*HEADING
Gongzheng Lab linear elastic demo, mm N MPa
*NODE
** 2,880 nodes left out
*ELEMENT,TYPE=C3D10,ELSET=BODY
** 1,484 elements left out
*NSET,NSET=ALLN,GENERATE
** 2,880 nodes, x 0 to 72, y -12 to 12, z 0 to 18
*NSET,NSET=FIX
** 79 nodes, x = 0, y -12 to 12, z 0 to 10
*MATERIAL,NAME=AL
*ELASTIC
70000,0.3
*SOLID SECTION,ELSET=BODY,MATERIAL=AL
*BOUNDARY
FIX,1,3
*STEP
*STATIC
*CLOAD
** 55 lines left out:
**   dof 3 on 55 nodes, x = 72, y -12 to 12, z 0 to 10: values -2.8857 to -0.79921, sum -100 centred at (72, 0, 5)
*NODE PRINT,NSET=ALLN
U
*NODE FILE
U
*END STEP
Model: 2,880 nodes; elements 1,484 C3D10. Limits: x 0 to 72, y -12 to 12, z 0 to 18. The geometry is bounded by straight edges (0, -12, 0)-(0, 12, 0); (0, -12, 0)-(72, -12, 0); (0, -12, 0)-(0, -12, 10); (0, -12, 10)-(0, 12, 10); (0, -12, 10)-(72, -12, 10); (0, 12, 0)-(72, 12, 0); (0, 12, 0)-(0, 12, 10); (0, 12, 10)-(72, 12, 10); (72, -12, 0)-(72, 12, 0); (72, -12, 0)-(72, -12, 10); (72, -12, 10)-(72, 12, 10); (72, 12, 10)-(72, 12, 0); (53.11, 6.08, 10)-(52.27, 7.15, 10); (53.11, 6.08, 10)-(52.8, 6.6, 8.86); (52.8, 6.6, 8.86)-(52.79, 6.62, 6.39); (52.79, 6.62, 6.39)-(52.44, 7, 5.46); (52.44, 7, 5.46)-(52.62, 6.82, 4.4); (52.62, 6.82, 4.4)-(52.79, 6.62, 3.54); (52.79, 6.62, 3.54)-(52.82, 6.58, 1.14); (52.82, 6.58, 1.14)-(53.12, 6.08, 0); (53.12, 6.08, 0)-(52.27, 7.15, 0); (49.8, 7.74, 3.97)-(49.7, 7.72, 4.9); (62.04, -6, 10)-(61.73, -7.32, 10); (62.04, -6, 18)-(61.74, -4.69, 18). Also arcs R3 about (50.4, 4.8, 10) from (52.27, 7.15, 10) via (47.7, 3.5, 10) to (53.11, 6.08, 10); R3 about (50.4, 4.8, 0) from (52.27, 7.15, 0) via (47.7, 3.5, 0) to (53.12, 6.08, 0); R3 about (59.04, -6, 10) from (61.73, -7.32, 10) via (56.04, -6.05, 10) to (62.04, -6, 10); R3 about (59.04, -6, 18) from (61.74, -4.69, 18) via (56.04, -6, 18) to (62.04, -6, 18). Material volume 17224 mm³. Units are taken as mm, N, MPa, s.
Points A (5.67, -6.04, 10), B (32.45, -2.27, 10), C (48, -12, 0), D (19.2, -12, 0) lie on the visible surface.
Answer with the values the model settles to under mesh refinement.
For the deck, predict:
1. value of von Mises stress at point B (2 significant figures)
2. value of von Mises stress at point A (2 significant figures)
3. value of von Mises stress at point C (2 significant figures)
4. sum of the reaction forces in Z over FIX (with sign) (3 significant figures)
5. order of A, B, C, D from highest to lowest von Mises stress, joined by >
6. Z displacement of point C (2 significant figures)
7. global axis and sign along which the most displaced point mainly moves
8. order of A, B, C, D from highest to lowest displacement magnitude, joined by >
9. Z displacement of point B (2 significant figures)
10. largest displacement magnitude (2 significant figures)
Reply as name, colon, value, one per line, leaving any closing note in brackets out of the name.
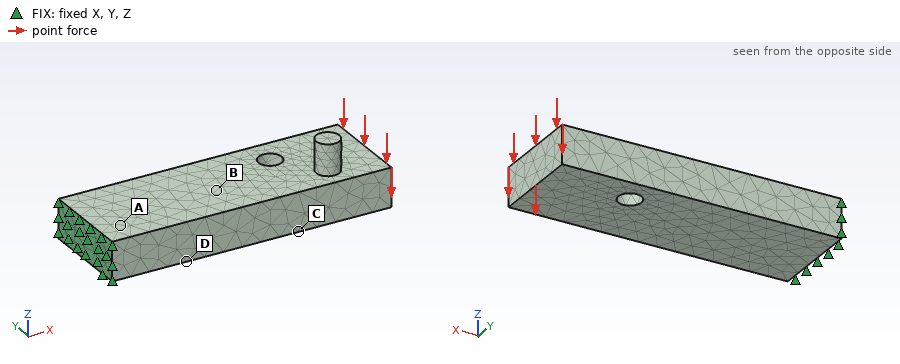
value of von Mises stress at point B: 9.9 MPa
value of von Mises stress at point A: 16 MPa
value of von Mises stress at point C: 6.8 MPa
sum of the reaction forces in Z over FIX (with sign): 100 N
order of A, B, C, D from highest to lowest von Mises stress, joined by >: A > D > B > C
Z displacement of point C: -0.046 mm
global axis and sign along which the most displaced point mainly moves: -Z
order of A, B, C, D from highest to lowest displacement magnitude, joined by >: C > B > D > A
Z displacement of point B: -0.023 mm
largest displacement magnitude: 0.090 mm
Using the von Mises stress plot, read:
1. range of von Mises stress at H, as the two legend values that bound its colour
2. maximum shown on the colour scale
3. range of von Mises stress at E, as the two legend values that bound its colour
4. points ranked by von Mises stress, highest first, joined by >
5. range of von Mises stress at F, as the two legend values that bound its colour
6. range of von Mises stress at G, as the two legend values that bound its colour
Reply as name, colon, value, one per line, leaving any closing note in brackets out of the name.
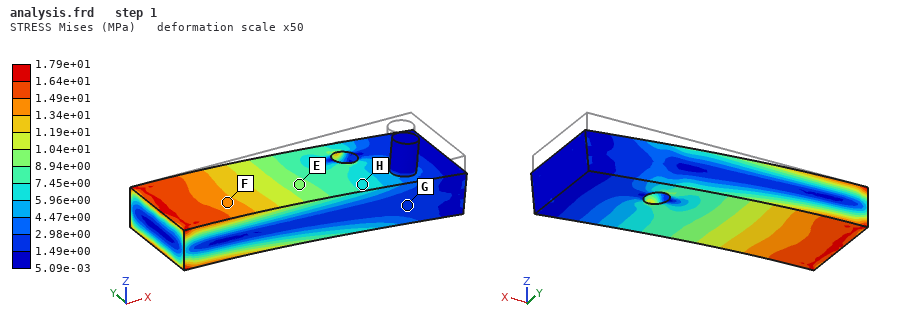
range of von Mises stress at H, as the two legend values that bound its colour: 5.96e+00 to 7.45e+00 MPa
maximum shown on the colour scale: 1.79e+01 MPa
range of von Mises stress at E, as the two legend values that bound its colour: 8.94e+00 to 1.04e+01 MPa
points ranked by von Mises stress, highest first, joined by >: F > E > H > G
range of von Mises stress at F, as the two legend values that bound its colour: 1.34e+01 to 1.49e+01 MPa
range of von Mises stress at G, as the two legend values that bound its colour: 1.49e+00 to 2.98e+00 MPa
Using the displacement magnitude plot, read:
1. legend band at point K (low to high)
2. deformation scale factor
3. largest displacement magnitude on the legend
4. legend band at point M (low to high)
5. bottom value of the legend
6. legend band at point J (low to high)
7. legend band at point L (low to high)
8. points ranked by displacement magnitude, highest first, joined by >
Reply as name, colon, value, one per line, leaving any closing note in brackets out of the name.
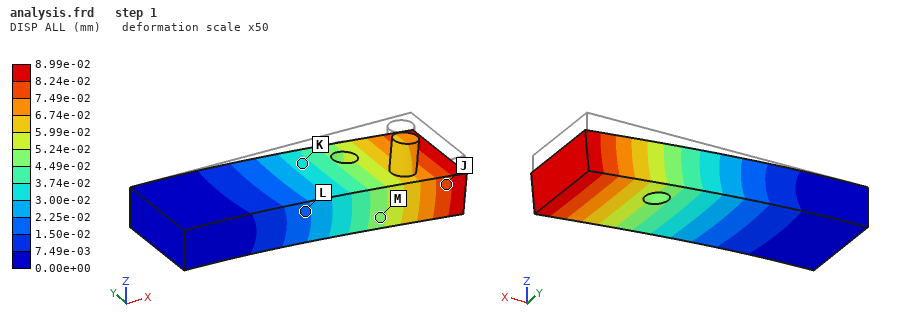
legend band at point K: 3.00e-02 to 3.74e-02 mm
deformation scale factor: 50
largest displacement magnitude on the legend: 8.99e-02 mm
legend band at point M: 4.49e-02 to 5.24e-02 mm
bottom value of the legend: 0.00e+00 mm
legend band at point J: 7.49e-02 to 8.24e-02 mm
legend band at point L: 1.50e-02 to 2.25e-02 mm
points ranked by displacement magnitude, highest first, joined by >: J > M > K > L
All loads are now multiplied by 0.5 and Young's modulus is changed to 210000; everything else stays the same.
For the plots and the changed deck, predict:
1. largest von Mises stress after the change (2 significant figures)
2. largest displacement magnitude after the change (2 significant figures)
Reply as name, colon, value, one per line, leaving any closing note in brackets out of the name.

largest von Mises stress after the change: 8.9 MPa
largest displacement magnitude after the change: 0.015 mm
